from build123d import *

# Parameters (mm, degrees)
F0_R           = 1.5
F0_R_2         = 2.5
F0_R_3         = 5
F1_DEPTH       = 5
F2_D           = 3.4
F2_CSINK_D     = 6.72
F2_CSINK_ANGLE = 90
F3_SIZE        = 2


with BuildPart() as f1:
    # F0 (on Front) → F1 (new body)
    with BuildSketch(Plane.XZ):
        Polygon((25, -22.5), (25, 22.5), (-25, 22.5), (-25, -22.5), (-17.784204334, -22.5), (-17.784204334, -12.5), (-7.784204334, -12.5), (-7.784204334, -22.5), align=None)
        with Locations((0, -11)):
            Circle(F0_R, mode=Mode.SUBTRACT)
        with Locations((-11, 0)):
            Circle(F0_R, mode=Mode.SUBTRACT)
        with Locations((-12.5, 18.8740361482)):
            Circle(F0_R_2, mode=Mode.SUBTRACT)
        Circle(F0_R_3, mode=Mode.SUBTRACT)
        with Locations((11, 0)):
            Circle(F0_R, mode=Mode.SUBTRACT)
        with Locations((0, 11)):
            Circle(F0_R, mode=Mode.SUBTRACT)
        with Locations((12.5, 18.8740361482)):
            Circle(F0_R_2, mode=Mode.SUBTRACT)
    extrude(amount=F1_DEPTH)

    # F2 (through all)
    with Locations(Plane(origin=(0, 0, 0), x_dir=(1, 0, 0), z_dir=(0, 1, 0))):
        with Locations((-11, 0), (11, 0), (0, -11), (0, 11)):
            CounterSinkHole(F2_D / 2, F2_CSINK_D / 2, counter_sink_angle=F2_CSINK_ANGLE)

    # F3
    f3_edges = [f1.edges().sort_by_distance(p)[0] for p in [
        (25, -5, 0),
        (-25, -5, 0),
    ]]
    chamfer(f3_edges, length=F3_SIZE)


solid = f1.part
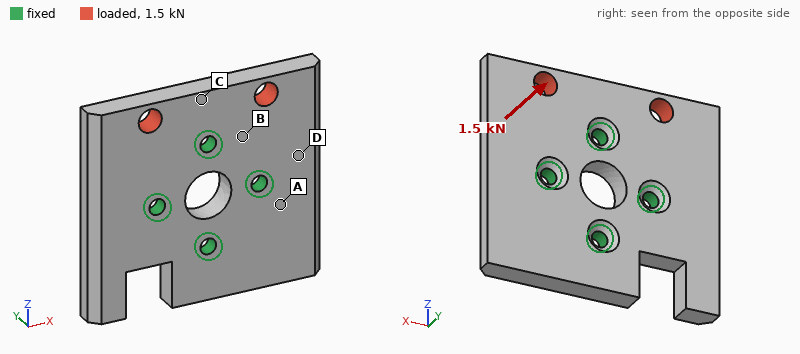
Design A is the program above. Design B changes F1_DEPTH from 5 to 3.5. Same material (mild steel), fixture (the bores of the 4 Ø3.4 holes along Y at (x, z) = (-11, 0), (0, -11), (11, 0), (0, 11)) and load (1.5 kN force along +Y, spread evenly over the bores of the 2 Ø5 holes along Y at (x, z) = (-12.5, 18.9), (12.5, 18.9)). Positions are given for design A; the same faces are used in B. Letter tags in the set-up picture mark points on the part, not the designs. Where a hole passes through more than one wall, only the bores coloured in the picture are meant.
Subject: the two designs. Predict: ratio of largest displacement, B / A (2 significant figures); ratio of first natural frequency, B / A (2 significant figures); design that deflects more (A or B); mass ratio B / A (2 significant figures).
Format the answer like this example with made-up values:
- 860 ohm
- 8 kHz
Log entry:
- 2.9
- 0.72
- B
- 0.69
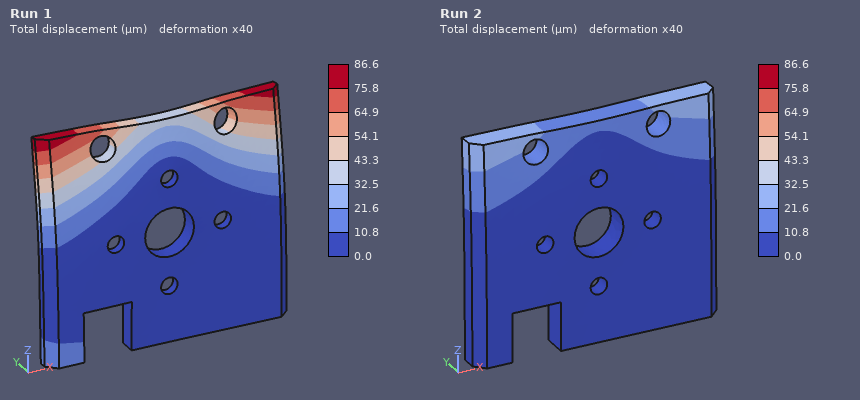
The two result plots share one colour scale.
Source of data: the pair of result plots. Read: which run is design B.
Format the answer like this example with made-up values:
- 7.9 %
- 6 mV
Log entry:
- Run 1
